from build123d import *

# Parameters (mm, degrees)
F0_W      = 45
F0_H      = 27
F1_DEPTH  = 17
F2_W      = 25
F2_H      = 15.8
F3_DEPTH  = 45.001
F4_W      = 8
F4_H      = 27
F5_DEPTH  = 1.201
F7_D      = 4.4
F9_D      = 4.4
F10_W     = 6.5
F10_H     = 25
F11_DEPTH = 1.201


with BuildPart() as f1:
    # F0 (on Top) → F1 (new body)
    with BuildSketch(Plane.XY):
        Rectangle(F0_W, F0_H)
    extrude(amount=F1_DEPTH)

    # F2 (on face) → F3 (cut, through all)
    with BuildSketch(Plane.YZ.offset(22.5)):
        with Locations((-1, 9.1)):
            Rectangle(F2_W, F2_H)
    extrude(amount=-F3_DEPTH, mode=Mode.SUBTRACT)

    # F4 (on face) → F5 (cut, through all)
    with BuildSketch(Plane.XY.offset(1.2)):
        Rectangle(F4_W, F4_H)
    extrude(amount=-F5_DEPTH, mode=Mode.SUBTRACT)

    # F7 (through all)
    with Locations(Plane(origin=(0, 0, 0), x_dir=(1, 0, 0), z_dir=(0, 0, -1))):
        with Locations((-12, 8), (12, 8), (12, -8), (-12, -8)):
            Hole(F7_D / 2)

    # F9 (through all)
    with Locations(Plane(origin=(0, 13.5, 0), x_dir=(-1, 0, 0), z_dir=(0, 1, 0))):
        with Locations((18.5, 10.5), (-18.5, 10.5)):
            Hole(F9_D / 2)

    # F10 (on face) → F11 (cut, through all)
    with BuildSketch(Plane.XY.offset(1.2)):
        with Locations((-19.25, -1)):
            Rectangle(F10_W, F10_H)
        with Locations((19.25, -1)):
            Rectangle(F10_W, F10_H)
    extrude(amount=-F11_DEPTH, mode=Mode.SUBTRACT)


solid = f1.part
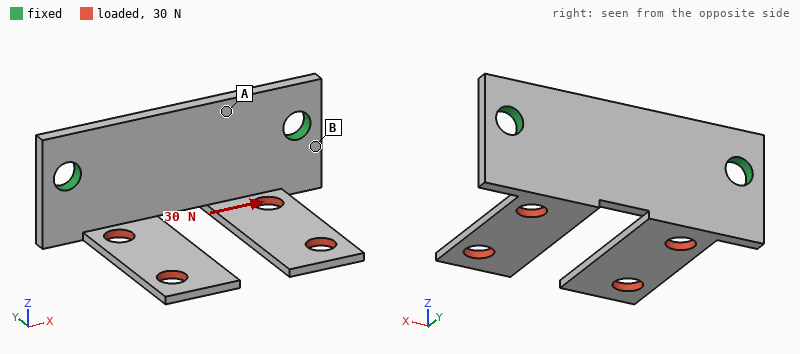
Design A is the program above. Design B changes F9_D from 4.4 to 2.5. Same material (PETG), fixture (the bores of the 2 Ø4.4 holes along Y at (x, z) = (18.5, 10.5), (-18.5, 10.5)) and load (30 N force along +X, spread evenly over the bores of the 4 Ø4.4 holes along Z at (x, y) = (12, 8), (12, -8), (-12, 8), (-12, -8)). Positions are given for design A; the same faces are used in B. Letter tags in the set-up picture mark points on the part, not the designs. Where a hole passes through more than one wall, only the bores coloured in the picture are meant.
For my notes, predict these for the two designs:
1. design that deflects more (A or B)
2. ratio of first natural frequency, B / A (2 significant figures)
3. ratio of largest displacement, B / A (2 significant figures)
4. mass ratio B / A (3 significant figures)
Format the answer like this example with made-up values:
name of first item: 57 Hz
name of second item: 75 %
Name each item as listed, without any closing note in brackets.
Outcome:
design that deflects more: B
ratio of first natural frequency, B / A: 0.98
ratio of largest displacement, B / A: 1.1
mass ratio B / A: 1.02
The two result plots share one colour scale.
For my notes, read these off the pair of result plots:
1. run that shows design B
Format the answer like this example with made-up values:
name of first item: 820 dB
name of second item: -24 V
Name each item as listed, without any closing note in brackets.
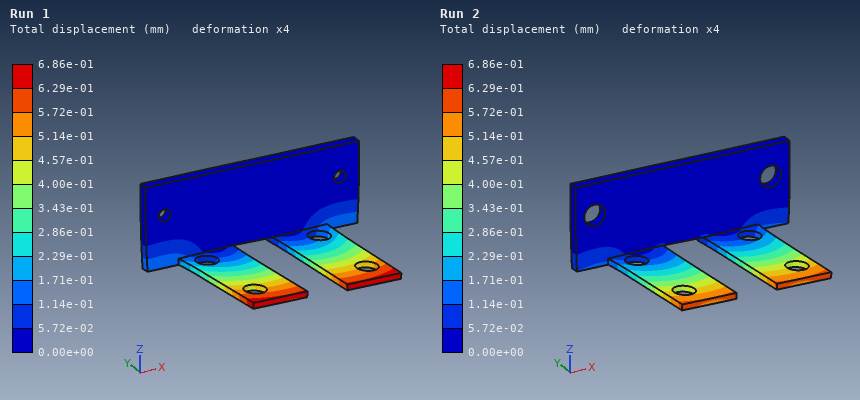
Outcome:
run that shows design B: Run 1
